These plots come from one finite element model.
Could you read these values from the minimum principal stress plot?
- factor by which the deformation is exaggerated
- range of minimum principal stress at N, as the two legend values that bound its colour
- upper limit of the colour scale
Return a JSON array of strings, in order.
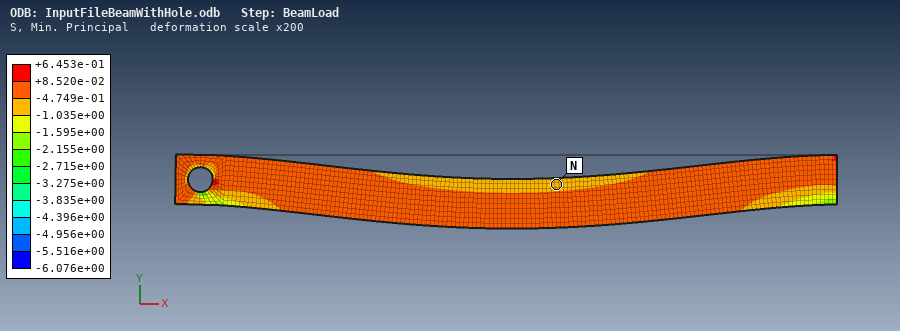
["200", "-1.035e+00 to -4.749e-01", "+6.453e-01"]
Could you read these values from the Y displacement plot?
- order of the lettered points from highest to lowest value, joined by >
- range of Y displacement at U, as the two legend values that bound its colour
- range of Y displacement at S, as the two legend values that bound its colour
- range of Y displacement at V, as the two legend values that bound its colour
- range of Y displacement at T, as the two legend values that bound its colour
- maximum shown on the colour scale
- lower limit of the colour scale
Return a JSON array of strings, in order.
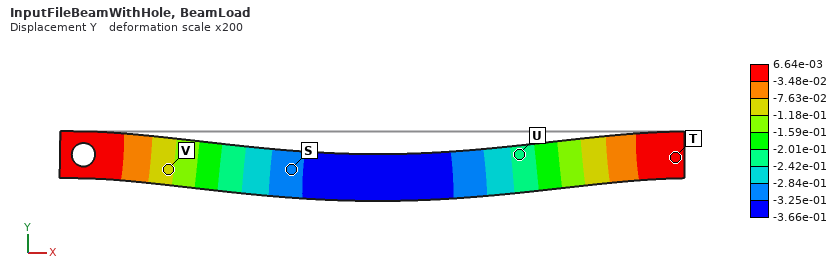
["T > V > U > S", "-2.42e-01 to -2.01e-01", "-3.25e-01 to -2.84e-01", "-1.18e-01 to -7.63e-02", "-3.48e-02 to 6.64e-03", "6.64e-03", "-3.66e-01"]
